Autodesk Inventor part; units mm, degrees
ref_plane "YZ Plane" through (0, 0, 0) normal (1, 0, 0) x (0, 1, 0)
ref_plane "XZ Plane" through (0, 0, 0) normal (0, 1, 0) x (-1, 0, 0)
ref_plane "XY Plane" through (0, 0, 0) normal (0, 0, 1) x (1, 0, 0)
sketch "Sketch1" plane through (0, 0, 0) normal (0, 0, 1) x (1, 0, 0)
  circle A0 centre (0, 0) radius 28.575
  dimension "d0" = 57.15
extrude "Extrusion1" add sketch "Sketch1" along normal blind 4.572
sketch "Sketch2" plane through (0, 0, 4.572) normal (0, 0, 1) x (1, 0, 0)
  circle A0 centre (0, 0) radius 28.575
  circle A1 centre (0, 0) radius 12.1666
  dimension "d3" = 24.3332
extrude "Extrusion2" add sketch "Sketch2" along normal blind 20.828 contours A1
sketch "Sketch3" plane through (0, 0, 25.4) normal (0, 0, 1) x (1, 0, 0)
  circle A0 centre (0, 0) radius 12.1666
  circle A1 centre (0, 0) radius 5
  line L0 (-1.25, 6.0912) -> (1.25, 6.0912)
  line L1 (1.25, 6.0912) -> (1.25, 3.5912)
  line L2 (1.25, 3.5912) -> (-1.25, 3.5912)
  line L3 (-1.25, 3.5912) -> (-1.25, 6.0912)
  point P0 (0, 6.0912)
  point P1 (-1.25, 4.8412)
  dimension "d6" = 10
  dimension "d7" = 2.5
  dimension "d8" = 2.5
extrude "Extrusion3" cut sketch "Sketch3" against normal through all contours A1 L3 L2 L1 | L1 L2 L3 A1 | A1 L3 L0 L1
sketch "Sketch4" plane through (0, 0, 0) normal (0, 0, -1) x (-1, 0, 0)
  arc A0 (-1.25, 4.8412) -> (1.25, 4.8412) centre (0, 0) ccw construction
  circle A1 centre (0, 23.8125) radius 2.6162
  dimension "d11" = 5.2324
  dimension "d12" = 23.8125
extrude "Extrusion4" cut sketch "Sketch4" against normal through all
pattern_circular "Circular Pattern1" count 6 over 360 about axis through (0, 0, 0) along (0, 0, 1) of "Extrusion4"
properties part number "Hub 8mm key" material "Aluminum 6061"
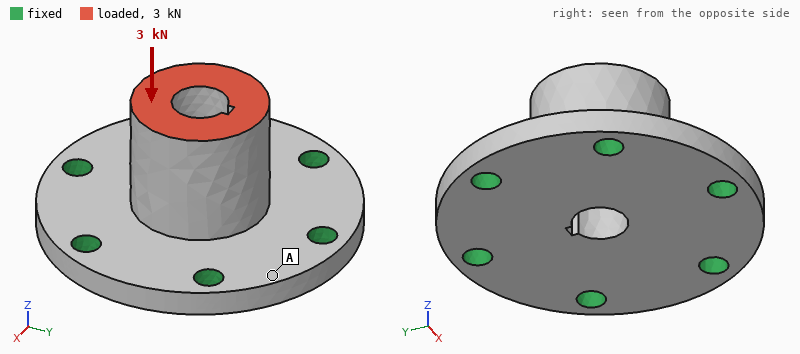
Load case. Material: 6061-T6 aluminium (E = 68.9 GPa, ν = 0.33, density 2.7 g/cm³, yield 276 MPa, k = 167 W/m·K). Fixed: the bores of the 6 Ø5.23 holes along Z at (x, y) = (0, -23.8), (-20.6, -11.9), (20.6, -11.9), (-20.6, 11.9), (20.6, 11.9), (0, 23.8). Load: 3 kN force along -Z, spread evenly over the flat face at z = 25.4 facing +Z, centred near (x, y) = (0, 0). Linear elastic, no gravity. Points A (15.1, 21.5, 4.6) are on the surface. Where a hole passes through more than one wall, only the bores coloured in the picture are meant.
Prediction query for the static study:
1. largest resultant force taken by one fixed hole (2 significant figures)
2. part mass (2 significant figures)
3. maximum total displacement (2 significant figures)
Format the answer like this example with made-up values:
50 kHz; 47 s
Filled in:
550 N; 51 g; 17 µm
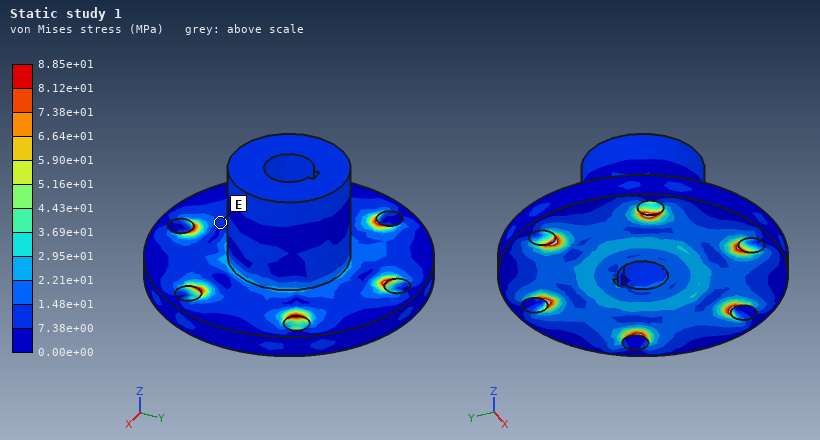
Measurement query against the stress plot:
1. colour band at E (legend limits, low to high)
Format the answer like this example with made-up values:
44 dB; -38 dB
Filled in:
7.38e+00 to 1.48e+01 MPa
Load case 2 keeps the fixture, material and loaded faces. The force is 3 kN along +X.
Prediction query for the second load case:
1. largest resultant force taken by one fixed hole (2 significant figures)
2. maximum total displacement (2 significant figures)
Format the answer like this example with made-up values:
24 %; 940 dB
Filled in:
1.3 kN; 72 µm
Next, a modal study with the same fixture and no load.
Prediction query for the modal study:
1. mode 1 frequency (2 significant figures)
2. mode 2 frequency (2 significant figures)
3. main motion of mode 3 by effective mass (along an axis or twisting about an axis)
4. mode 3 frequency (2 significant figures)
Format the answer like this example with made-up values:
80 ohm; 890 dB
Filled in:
11 kHz; 11 kHz; along Z; 13 kHz
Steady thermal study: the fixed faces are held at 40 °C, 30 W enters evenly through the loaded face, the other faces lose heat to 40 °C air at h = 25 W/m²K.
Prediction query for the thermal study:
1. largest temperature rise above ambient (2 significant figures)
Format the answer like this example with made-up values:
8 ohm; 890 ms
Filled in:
15 K
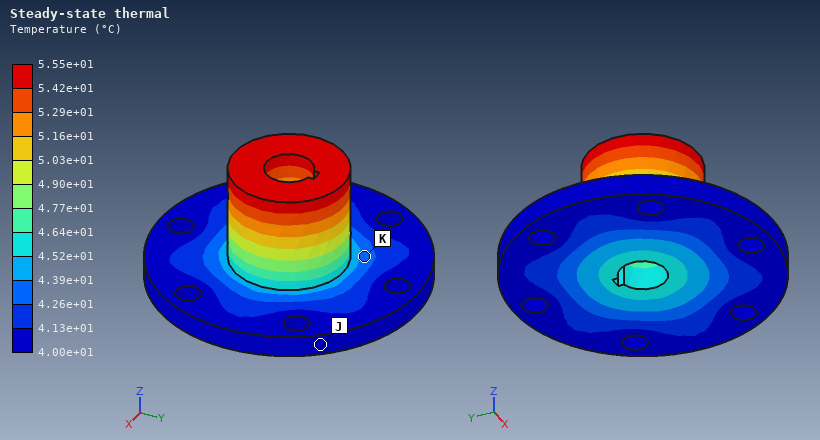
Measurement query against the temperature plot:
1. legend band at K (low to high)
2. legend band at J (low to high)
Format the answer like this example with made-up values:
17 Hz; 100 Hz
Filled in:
4.26e+01 to 4.39e+01 °C; 4.00e+01 to 4.13e+01 °C
